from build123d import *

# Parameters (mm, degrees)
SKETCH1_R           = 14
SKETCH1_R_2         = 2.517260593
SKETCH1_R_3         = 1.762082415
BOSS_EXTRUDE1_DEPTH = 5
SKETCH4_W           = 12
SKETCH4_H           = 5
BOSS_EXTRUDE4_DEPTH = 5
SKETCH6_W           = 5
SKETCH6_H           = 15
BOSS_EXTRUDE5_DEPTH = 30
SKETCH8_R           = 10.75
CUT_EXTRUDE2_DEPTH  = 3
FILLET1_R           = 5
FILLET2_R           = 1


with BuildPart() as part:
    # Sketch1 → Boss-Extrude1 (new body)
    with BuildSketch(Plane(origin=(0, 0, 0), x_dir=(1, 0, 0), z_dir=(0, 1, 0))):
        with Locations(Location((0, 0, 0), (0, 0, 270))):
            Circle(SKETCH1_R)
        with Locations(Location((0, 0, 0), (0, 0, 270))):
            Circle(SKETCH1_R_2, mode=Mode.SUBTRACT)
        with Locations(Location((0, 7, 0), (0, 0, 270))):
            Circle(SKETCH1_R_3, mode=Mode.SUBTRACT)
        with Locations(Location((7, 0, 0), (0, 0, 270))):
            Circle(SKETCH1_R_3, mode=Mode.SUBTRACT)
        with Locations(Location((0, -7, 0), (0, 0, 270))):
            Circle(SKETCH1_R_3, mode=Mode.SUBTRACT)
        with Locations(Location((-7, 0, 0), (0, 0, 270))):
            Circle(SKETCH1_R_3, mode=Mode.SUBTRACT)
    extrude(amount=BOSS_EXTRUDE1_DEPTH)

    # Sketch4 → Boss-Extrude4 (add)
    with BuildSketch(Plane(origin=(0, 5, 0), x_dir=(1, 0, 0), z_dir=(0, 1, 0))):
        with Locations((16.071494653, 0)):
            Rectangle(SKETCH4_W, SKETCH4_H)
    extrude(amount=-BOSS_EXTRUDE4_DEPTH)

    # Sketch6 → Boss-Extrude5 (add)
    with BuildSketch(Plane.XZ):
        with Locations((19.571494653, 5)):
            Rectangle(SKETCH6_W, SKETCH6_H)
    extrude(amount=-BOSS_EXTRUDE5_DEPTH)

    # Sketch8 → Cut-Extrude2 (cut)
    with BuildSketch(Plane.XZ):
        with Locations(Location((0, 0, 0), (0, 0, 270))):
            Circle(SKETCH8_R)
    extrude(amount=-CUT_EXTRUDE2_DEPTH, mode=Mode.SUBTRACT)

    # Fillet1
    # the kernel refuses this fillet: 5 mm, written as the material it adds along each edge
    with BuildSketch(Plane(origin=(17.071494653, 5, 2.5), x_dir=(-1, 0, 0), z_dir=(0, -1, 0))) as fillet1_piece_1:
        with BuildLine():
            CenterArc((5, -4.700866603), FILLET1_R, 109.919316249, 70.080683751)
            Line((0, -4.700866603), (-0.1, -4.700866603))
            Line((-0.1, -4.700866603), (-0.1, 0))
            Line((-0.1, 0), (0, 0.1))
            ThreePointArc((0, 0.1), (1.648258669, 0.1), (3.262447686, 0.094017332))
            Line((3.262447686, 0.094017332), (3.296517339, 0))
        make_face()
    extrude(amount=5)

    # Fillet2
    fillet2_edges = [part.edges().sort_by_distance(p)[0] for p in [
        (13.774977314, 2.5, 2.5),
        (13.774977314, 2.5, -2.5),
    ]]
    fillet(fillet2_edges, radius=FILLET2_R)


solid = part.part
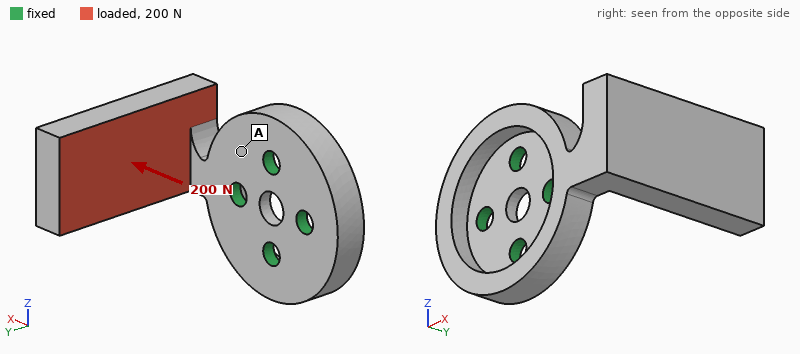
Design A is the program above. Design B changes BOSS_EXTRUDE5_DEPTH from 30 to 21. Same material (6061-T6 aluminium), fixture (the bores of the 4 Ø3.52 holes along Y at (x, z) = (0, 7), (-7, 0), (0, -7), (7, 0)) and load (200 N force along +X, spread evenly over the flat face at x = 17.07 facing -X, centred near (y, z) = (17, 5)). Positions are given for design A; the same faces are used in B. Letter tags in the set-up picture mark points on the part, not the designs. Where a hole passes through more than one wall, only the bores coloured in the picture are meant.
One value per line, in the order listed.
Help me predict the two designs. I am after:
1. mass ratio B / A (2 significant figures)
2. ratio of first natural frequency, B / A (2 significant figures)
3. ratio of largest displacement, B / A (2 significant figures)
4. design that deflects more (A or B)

0.84
1.6
0.47
A
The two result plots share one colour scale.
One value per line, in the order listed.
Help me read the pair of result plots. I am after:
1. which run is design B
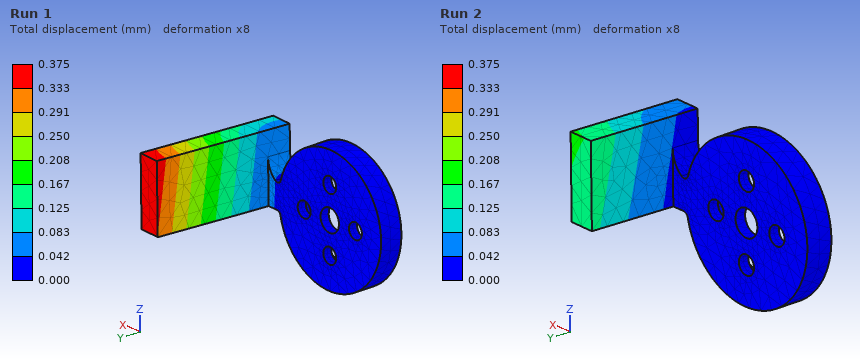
Run 2
